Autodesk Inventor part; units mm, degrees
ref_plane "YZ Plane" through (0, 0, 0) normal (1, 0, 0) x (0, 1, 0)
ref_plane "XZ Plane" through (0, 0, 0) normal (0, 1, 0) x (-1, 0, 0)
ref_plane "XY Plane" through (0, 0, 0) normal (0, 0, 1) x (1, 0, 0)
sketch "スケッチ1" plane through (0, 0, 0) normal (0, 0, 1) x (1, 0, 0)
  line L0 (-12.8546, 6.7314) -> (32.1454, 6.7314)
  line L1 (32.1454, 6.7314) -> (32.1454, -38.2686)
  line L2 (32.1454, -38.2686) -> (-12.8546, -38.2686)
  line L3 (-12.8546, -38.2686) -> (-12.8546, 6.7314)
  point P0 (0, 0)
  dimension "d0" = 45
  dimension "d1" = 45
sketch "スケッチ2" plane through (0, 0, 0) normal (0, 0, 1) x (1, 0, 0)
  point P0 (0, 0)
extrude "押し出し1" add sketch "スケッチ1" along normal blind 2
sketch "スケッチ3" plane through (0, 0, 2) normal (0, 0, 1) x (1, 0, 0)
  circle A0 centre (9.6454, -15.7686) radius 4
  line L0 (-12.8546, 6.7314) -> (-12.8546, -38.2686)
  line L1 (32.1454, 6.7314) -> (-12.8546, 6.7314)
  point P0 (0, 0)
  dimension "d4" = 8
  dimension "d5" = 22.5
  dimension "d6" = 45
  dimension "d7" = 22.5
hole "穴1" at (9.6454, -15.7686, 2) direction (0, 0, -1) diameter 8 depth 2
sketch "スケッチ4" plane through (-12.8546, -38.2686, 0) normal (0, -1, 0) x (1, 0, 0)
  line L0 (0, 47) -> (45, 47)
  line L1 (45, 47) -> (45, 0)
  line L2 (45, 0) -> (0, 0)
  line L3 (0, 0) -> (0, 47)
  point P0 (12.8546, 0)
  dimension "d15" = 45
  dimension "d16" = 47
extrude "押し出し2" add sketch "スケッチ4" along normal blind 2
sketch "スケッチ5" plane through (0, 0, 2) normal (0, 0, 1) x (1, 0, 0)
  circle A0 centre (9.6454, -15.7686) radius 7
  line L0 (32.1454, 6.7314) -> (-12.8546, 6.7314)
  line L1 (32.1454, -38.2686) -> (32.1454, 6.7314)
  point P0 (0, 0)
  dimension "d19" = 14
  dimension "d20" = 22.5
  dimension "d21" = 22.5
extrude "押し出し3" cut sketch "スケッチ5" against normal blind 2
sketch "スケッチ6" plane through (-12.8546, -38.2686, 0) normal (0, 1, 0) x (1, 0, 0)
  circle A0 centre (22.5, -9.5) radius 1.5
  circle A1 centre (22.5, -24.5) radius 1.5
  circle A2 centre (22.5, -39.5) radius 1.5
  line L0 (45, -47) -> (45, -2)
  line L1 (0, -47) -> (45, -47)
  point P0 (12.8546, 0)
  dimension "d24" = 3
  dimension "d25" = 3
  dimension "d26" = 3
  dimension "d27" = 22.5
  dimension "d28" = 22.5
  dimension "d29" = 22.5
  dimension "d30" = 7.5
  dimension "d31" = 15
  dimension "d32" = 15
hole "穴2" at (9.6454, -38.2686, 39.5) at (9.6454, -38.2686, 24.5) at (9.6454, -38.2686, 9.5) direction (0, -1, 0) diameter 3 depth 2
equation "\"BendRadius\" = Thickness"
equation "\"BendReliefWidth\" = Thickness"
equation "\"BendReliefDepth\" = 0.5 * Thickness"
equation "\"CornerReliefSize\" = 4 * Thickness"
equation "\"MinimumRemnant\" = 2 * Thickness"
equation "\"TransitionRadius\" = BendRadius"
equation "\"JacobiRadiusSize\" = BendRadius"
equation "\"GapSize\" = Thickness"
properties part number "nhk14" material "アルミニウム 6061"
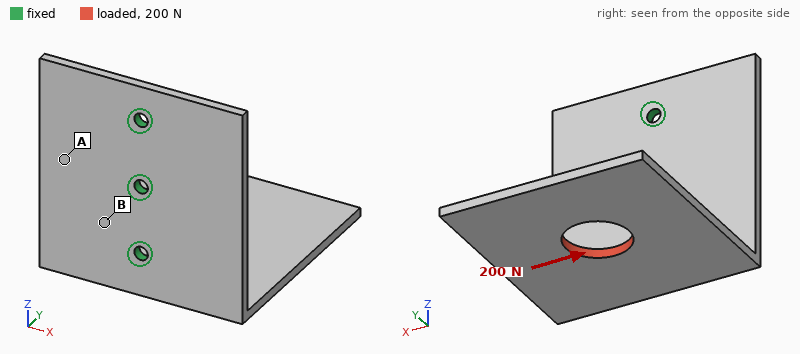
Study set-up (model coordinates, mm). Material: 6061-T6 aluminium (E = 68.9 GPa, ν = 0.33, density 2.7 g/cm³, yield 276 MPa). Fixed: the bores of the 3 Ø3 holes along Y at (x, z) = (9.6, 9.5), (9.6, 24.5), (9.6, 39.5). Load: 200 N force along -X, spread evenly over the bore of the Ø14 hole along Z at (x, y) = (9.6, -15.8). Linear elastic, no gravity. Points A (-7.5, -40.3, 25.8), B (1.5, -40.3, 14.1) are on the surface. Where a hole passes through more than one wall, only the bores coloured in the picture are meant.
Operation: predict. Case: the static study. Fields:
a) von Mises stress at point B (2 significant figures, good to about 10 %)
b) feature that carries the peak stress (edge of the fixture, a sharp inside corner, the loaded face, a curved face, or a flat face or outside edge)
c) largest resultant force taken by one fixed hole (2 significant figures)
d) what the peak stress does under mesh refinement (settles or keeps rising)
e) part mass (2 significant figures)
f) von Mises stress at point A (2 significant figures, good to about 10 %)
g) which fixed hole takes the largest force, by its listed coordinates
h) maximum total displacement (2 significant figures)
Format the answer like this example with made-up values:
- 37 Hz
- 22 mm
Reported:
- 71 MPa
- edge of the fixture
- 230 N
- keeps rising
- 21 g
- 35 MPa
- (9.6, 9.5)
- 0.76 mm
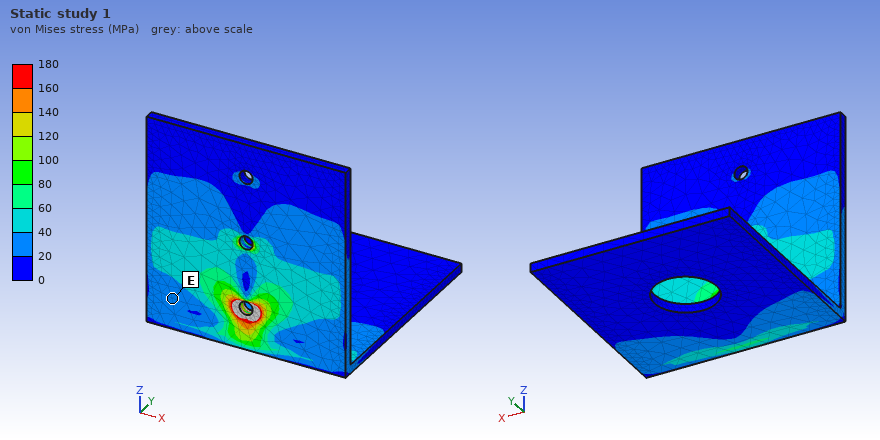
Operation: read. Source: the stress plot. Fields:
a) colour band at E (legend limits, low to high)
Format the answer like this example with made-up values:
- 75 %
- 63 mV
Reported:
- 20 to 40 MPa
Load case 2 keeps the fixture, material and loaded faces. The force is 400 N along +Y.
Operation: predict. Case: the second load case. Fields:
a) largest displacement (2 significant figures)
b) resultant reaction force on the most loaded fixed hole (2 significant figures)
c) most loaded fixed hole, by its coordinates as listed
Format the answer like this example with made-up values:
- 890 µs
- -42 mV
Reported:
- 0.45 mm
- 480 N
- (9.6, 9.5)
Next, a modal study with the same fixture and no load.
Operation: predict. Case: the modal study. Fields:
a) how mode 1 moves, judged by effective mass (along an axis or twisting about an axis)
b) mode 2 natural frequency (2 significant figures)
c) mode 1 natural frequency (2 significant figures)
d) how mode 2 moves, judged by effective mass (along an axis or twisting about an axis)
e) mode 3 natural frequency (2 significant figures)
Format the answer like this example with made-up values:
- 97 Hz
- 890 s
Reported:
- along Z
- 910 Hz
- 580 Hz
- along X
- 1700 Hz
